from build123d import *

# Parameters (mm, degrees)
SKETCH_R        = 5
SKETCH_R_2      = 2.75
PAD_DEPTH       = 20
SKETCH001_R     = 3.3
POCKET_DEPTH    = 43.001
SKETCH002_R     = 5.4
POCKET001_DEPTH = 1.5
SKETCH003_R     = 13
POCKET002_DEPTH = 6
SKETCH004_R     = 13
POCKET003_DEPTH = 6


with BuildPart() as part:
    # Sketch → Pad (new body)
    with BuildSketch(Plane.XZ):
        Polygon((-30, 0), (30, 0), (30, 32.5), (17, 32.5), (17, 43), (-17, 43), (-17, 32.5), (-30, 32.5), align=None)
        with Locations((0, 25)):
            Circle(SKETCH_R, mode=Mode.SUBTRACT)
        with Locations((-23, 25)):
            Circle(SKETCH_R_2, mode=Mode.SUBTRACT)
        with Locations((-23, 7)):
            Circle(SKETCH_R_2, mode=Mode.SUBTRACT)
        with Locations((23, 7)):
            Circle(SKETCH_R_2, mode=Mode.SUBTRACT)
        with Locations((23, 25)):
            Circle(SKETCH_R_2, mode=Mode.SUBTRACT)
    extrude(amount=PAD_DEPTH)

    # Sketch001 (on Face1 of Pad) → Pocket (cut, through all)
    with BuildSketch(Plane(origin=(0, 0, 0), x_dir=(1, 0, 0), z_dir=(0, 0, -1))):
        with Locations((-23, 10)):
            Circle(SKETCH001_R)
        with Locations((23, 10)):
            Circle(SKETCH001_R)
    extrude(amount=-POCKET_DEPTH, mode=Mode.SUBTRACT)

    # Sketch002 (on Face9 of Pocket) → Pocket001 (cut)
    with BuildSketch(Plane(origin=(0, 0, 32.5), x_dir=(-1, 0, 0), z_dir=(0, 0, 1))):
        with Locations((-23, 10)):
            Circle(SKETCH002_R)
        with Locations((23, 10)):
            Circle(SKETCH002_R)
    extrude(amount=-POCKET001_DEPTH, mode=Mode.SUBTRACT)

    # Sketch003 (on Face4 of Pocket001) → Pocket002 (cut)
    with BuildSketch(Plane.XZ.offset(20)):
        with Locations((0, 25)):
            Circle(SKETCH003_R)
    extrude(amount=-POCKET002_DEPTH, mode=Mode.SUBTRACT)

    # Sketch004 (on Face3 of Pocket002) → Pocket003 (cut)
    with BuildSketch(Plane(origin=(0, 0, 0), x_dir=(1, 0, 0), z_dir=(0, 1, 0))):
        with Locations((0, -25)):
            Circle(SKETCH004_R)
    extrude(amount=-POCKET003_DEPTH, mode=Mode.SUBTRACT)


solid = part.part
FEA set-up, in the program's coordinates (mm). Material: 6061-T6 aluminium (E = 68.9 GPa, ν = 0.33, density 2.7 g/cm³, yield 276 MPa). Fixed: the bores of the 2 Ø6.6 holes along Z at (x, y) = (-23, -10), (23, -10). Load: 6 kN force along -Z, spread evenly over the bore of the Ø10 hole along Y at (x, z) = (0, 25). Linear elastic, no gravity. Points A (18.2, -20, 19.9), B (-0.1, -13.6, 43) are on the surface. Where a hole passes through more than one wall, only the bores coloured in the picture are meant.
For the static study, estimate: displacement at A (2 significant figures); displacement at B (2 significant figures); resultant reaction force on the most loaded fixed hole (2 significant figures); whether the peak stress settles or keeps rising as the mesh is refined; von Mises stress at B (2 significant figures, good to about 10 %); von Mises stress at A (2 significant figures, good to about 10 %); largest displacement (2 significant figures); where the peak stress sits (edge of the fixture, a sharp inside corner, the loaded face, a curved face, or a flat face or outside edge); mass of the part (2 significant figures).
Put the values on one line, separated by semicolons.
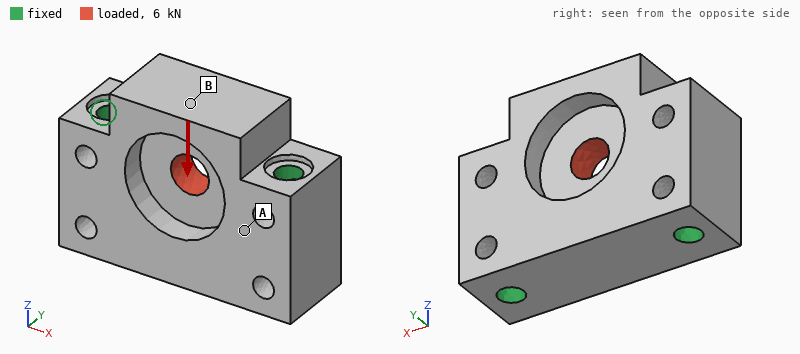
1.2 µm; 5.2 µm; 3.1 kN; keeps rising; 15 MPa; 5.4 MPa; 7.9 µm; edge of the fixture; 96 g
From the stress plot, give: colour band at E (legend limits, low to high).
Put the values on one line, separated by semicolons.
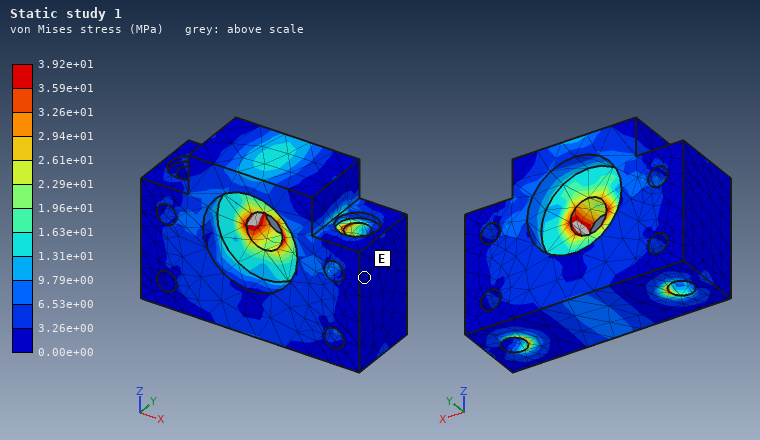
0.00e+00 to 3.26e+00 MPa
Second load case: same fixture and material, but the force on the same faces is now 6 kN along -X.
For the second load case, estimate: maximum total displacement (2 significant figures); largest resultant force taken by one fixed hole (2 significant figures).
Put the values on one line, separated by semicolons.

5.6 µm; 3.0 kN
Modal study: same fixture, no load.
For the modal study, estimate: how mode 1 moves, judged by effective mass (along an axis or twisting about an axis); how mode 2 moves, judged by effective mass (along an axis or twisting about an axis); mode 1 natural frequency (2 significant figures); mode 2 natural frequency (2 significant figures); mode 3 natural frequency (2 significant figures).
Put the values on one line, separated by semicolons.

along Y; along Y; 15 kHz; 25 kHz; 27 kHz
